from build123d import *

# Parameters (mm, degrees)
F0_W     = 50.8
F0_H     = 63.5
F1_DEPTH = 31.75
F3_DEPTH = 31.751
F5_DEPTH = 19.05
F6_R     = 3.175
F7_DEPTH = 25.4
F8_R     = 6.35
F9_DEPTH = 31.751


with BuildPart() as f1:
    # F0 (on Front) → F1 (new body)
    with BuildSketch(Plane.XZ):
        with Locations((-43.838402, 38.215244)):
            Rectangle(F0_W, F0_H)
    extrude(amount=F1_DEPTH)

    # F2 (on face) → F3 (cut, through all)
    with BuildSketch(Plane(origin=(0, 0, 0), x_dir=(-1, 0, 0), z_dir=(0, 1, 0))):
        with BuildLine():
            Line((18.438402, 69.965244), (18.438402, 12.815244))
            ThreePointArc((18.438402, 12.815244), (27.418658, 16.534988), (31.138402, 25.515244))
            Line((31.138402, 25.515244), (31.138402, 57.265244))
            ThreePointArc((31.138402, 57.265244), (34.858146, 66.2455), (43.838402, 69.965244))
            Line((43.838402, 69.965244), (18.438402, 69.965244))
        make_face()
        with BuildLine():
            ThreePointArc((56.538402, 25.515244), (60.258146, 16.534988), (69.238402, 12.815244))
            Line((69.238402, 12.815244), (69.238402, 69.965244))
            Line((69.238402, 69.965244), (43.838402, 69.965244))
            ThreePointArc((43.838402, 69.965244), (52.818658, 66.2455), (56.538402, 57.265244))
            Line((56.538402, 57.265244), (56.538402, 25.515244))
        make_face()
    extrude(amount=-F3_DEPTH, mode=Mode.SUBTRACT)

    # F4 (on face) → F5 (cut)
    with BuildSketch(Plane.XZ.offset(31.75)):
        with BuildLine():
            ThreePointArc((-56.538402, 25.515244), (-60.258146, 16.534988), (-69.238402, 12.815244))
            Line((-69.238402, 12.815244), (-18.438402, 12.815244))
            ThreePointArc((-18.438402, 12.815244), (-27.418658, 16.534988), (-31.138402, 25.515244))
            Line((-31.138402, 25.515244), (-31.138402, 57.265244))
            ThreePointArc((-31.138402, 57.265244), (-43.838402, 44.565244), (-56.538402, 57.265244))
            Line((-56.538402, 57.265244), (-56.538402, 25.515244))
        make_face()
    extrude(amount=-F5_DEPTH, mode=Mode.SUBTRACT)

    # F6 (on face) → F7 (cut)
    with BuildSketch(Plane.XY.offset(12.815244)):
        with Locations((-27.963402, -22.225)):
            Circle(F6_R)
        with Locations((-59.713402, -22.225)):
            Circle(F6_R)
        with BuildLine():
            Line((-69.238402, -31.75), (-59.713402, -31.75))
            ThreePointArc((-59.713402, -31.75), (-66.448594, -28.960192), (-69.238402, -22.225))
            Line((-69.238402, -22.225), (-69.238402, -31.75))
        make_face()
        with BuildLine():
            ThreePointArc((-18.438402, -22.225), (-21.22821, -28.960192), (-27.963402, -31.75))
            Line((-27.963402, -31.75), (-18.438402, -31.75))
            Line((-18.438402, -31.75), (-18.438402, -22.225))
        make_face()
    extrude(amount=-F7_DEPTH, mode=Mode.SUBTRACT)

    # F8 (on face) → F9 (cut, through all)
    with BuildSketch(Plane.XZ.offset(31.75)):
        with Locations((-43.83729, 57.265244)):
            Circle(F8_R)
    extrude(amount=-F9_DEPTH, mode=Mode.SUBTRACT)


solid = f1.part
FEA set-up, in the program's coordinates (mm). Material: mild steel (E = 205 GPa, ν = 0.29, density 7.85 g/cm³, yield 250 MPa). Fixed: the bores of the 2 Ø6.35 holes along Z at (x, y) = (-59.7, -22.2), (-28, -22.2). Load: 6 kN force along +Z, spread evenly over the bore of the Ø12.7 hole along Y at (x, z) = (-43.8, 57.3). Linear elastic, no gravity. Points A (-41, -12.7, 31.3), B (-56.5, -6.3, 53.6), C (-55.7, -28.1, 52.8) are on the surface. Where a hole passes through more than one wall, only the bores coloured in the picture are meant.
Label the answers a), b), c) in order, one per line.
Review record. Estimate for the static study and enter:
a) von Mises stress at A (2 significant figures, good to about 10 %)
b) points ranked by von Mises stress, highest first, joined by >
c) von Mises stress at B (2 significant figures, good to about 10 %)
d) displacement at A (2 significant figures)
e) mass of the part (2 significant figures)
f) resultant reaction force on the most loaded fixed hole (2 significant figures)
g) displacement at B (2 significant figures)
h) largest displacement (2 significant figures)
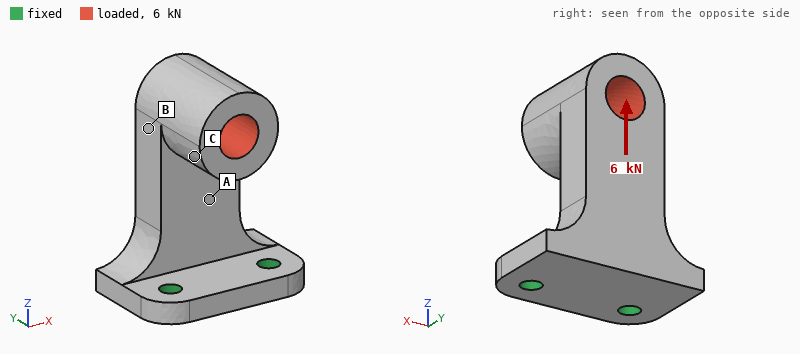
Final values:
a) 97 MPa
b) A > B > C
c) 31 MPa
d) 0.021 mm
e) 260 g
f) 3.0 kN
g) 0.055 mm
h) 0.13 mm
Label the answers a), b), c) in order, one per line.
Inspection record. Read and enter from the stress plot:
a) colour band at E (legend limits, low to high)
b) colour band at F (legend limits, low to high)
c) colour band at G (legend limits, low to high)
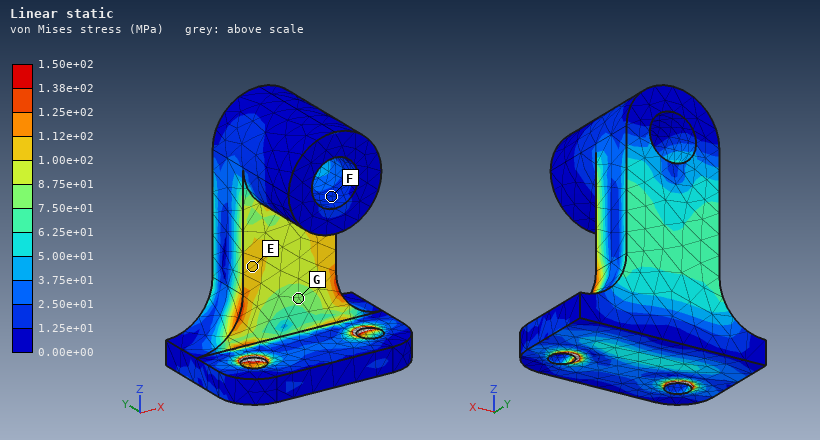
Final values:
a) 1.00e+02 to 1.12e+02 MPa
b) 1.25e+01 to 2.50e+01 MPa
c) 7.50e+01 to 8.75e+01 MPa
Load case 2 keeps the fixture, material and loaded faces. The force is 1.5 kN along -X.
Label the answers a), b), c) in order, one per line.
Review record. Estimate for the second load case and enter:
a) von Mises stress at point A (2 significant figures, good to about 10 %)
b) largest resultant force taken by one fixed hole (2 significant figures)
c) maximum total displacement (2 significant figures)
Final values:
a) 39 MPa
b) 2.3 kN
c) 74 µm
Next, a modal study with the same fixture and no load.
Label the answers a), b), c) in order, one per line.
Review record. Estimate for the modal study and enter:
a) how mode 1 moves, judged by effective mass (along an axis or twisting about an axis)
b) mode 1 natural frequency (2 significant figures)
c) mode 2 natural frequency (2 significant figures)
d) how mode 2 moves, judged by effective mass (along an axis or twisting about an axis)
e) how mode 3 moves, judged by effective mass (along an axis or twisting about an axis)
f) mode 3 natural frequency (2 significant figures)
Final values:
a) along Y
b) 1100 Hz
c) 2600 Hz
d) along X
e) along Z
f) 5200 Hz
